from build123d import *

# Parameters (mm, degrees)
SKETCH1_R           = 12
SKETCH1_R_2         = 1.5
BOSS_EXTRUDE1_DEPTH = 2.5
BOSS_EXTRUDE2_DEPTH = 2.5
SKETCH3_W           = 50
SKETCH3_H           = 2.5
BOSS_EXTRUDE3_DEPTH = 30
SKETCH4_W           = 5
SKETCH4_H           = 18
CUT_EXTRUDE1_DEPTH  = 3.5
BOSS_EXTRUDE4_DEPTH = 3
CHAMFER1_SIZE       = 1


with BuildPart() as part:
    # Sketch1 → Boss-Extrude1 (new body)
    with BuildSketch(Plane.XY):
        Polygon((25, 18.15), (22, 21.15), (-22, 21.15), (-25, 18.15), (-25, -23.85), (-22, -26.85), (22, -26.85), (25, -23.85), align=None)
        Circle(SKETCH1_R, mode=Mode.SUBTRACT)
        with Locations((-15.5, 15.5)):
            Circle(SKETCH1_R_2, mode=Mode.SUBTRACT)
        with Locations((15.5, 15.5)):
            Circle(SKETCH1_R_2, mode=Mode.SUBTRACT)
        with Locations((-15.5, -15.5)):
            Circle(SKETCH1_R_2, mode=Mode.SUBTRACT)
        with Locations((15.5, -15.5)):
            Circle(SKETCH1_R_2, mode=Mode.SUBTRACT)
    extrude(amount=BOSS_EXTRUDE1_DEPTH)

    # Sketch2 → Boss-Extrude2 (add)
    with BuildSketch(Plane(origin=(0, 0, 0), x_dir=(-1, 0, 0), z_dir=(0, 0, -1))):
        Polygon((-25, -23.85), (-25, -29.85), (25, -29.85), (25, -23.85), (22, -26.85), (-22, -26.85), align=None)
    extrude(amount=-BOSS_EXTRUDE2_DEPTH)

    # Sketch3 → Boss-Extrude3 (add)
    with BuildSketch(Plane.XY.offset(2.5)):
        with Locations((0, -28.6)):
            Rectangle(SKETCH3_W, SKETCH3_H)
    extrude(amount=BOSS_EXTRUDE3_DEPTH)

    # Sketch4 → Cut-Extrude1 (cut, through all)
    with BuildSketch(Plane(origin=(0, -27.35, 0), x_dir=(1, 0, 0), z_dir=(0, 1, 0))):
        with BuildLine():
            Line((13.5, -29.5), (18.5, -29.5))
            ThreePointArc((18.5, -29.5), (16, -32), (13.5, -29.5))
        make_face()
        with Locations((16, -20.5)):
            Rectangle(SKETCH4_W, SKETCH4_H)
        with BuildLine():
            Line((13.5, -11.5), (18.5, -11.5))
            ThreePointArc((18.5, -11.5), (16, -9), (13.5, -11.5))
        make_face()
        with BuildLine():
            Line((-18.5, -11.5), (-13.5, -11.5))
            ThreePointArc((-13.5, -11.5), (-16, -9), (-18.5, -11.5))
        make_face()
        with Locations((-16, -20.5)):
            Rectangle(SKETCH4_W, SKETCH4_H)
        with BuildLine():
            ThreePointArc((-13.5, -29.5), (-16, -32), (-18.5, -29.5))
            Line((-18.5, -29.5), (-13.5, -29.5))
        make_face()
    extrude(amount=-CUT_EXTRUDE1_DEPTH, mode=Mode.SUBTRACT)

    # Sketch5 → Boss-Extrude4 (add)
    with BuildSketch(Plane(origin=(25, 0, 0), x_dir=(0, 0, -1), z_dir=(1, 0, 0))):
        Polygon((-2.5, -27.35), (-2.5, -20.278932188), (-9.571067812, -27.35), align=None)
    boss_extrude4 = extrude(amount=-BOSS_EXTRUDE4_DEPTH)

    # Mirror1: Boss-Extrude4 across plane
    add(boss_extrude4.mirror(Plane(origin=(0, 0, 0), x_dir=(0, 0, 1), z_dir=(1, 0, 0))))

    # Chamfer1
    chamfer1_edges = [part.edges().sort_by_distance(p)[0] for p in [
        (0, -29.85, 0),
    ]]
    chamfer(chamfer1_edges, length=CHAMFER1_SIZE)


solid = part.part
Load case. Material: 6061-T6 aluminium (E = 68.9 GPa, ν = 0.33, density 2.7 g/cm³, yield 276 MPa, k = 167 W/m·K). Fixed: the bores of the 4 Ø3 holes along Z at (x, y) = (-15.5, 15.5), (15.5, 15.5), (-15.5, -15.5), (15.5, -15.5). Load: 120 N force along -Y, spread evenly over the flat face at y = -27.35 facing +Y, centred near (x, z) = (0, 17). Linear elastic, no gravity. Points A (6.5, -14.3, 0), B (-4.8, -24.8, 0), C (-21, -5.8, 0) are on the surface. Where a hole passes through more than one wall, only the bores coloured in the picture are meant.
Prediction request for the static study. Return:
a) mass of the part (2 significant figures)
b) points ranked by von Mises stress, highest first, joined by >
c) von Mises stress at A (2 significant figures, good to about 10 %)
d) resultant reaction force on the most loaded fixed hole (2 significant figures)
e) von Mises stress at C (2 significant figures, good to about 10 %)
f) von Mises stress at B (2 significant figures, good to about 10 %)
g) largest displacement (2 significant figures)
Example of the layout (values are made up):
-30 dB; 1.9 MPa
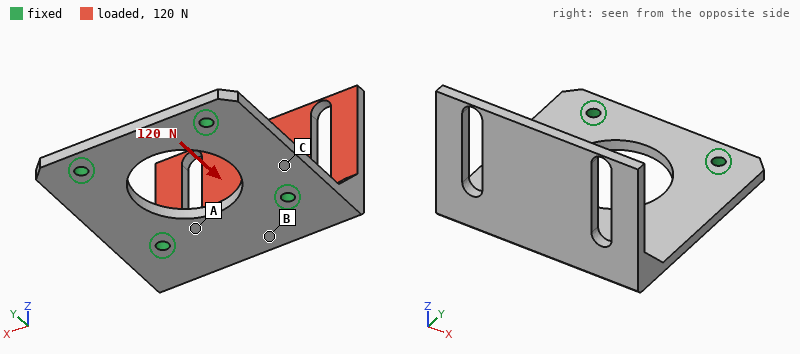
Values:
23 g; B > A > C; 15 MPa; 56 N; 6.3 MPa; 26 MPa; 0.24 mm
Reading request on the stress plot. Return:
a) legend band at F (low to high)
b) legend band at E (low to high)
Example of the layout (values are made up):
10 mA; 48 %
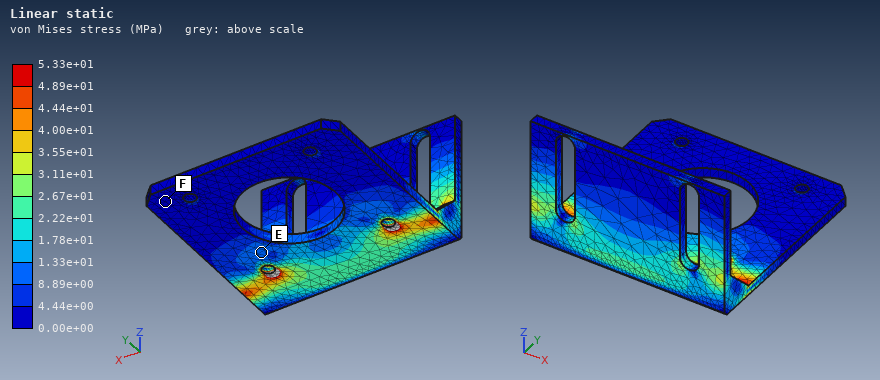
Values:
0.00e+00 to 4.44e+00 MPa; 8.89e+00 to 1.33e+01 MPa
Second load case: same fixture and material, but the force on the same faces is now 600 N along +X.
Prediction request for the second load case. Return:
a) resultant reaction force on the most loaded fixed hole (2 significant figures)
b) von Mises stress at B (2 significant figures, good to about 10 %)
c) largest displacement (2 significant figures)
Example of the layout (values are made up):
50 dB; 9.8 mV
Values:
450 N; 37 MPa; 0.24 mm
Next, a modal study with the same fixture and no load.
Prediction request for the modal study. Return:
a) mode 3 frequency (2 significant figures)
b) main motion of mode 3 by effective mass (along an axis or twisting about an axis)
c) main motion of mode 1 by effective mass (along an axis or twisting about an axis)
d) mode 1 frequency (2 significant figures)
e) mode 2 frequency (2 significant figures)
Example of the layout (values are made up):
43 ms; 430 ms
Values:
4800 Hz; along Z; along Y; 1500 Hz; 2800 Hz
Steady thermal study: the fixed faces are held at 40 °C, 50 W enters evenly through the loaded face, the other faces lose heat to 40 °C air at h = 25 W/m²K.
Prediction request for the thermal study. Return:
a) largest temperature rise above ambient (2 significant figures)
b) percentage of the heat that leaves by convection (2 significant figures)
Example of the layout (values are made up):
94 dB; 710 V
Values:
76 K; 8.0 %
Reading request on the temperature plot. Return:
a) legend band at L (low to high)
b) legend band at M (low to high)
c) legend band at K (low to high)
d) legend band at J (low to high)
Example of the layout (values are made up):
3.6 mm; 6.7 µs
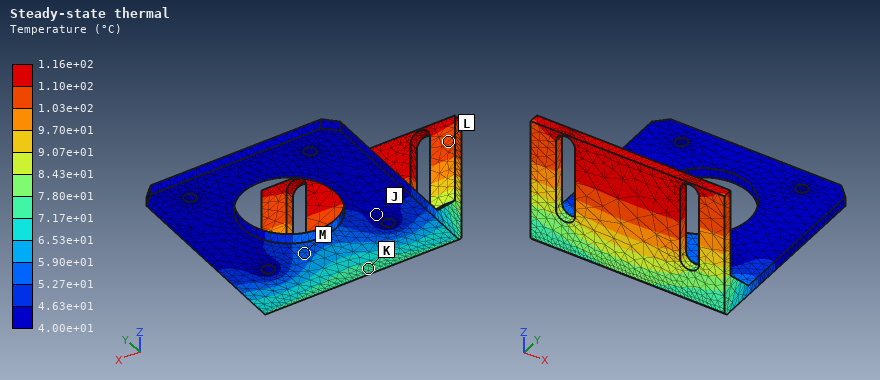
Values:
1.03e+02 to 1.10e+02 °C; 5.27e+01 to 5.90e+01 °C; 7.17e+01 to 7.80e+01 °C; 4.00e+01 to 4.63e+01 °C
